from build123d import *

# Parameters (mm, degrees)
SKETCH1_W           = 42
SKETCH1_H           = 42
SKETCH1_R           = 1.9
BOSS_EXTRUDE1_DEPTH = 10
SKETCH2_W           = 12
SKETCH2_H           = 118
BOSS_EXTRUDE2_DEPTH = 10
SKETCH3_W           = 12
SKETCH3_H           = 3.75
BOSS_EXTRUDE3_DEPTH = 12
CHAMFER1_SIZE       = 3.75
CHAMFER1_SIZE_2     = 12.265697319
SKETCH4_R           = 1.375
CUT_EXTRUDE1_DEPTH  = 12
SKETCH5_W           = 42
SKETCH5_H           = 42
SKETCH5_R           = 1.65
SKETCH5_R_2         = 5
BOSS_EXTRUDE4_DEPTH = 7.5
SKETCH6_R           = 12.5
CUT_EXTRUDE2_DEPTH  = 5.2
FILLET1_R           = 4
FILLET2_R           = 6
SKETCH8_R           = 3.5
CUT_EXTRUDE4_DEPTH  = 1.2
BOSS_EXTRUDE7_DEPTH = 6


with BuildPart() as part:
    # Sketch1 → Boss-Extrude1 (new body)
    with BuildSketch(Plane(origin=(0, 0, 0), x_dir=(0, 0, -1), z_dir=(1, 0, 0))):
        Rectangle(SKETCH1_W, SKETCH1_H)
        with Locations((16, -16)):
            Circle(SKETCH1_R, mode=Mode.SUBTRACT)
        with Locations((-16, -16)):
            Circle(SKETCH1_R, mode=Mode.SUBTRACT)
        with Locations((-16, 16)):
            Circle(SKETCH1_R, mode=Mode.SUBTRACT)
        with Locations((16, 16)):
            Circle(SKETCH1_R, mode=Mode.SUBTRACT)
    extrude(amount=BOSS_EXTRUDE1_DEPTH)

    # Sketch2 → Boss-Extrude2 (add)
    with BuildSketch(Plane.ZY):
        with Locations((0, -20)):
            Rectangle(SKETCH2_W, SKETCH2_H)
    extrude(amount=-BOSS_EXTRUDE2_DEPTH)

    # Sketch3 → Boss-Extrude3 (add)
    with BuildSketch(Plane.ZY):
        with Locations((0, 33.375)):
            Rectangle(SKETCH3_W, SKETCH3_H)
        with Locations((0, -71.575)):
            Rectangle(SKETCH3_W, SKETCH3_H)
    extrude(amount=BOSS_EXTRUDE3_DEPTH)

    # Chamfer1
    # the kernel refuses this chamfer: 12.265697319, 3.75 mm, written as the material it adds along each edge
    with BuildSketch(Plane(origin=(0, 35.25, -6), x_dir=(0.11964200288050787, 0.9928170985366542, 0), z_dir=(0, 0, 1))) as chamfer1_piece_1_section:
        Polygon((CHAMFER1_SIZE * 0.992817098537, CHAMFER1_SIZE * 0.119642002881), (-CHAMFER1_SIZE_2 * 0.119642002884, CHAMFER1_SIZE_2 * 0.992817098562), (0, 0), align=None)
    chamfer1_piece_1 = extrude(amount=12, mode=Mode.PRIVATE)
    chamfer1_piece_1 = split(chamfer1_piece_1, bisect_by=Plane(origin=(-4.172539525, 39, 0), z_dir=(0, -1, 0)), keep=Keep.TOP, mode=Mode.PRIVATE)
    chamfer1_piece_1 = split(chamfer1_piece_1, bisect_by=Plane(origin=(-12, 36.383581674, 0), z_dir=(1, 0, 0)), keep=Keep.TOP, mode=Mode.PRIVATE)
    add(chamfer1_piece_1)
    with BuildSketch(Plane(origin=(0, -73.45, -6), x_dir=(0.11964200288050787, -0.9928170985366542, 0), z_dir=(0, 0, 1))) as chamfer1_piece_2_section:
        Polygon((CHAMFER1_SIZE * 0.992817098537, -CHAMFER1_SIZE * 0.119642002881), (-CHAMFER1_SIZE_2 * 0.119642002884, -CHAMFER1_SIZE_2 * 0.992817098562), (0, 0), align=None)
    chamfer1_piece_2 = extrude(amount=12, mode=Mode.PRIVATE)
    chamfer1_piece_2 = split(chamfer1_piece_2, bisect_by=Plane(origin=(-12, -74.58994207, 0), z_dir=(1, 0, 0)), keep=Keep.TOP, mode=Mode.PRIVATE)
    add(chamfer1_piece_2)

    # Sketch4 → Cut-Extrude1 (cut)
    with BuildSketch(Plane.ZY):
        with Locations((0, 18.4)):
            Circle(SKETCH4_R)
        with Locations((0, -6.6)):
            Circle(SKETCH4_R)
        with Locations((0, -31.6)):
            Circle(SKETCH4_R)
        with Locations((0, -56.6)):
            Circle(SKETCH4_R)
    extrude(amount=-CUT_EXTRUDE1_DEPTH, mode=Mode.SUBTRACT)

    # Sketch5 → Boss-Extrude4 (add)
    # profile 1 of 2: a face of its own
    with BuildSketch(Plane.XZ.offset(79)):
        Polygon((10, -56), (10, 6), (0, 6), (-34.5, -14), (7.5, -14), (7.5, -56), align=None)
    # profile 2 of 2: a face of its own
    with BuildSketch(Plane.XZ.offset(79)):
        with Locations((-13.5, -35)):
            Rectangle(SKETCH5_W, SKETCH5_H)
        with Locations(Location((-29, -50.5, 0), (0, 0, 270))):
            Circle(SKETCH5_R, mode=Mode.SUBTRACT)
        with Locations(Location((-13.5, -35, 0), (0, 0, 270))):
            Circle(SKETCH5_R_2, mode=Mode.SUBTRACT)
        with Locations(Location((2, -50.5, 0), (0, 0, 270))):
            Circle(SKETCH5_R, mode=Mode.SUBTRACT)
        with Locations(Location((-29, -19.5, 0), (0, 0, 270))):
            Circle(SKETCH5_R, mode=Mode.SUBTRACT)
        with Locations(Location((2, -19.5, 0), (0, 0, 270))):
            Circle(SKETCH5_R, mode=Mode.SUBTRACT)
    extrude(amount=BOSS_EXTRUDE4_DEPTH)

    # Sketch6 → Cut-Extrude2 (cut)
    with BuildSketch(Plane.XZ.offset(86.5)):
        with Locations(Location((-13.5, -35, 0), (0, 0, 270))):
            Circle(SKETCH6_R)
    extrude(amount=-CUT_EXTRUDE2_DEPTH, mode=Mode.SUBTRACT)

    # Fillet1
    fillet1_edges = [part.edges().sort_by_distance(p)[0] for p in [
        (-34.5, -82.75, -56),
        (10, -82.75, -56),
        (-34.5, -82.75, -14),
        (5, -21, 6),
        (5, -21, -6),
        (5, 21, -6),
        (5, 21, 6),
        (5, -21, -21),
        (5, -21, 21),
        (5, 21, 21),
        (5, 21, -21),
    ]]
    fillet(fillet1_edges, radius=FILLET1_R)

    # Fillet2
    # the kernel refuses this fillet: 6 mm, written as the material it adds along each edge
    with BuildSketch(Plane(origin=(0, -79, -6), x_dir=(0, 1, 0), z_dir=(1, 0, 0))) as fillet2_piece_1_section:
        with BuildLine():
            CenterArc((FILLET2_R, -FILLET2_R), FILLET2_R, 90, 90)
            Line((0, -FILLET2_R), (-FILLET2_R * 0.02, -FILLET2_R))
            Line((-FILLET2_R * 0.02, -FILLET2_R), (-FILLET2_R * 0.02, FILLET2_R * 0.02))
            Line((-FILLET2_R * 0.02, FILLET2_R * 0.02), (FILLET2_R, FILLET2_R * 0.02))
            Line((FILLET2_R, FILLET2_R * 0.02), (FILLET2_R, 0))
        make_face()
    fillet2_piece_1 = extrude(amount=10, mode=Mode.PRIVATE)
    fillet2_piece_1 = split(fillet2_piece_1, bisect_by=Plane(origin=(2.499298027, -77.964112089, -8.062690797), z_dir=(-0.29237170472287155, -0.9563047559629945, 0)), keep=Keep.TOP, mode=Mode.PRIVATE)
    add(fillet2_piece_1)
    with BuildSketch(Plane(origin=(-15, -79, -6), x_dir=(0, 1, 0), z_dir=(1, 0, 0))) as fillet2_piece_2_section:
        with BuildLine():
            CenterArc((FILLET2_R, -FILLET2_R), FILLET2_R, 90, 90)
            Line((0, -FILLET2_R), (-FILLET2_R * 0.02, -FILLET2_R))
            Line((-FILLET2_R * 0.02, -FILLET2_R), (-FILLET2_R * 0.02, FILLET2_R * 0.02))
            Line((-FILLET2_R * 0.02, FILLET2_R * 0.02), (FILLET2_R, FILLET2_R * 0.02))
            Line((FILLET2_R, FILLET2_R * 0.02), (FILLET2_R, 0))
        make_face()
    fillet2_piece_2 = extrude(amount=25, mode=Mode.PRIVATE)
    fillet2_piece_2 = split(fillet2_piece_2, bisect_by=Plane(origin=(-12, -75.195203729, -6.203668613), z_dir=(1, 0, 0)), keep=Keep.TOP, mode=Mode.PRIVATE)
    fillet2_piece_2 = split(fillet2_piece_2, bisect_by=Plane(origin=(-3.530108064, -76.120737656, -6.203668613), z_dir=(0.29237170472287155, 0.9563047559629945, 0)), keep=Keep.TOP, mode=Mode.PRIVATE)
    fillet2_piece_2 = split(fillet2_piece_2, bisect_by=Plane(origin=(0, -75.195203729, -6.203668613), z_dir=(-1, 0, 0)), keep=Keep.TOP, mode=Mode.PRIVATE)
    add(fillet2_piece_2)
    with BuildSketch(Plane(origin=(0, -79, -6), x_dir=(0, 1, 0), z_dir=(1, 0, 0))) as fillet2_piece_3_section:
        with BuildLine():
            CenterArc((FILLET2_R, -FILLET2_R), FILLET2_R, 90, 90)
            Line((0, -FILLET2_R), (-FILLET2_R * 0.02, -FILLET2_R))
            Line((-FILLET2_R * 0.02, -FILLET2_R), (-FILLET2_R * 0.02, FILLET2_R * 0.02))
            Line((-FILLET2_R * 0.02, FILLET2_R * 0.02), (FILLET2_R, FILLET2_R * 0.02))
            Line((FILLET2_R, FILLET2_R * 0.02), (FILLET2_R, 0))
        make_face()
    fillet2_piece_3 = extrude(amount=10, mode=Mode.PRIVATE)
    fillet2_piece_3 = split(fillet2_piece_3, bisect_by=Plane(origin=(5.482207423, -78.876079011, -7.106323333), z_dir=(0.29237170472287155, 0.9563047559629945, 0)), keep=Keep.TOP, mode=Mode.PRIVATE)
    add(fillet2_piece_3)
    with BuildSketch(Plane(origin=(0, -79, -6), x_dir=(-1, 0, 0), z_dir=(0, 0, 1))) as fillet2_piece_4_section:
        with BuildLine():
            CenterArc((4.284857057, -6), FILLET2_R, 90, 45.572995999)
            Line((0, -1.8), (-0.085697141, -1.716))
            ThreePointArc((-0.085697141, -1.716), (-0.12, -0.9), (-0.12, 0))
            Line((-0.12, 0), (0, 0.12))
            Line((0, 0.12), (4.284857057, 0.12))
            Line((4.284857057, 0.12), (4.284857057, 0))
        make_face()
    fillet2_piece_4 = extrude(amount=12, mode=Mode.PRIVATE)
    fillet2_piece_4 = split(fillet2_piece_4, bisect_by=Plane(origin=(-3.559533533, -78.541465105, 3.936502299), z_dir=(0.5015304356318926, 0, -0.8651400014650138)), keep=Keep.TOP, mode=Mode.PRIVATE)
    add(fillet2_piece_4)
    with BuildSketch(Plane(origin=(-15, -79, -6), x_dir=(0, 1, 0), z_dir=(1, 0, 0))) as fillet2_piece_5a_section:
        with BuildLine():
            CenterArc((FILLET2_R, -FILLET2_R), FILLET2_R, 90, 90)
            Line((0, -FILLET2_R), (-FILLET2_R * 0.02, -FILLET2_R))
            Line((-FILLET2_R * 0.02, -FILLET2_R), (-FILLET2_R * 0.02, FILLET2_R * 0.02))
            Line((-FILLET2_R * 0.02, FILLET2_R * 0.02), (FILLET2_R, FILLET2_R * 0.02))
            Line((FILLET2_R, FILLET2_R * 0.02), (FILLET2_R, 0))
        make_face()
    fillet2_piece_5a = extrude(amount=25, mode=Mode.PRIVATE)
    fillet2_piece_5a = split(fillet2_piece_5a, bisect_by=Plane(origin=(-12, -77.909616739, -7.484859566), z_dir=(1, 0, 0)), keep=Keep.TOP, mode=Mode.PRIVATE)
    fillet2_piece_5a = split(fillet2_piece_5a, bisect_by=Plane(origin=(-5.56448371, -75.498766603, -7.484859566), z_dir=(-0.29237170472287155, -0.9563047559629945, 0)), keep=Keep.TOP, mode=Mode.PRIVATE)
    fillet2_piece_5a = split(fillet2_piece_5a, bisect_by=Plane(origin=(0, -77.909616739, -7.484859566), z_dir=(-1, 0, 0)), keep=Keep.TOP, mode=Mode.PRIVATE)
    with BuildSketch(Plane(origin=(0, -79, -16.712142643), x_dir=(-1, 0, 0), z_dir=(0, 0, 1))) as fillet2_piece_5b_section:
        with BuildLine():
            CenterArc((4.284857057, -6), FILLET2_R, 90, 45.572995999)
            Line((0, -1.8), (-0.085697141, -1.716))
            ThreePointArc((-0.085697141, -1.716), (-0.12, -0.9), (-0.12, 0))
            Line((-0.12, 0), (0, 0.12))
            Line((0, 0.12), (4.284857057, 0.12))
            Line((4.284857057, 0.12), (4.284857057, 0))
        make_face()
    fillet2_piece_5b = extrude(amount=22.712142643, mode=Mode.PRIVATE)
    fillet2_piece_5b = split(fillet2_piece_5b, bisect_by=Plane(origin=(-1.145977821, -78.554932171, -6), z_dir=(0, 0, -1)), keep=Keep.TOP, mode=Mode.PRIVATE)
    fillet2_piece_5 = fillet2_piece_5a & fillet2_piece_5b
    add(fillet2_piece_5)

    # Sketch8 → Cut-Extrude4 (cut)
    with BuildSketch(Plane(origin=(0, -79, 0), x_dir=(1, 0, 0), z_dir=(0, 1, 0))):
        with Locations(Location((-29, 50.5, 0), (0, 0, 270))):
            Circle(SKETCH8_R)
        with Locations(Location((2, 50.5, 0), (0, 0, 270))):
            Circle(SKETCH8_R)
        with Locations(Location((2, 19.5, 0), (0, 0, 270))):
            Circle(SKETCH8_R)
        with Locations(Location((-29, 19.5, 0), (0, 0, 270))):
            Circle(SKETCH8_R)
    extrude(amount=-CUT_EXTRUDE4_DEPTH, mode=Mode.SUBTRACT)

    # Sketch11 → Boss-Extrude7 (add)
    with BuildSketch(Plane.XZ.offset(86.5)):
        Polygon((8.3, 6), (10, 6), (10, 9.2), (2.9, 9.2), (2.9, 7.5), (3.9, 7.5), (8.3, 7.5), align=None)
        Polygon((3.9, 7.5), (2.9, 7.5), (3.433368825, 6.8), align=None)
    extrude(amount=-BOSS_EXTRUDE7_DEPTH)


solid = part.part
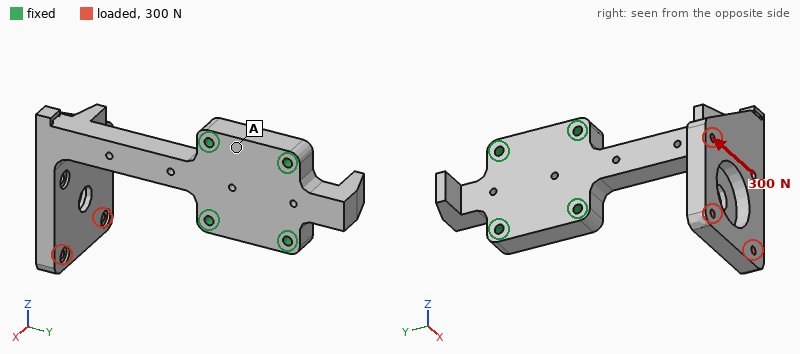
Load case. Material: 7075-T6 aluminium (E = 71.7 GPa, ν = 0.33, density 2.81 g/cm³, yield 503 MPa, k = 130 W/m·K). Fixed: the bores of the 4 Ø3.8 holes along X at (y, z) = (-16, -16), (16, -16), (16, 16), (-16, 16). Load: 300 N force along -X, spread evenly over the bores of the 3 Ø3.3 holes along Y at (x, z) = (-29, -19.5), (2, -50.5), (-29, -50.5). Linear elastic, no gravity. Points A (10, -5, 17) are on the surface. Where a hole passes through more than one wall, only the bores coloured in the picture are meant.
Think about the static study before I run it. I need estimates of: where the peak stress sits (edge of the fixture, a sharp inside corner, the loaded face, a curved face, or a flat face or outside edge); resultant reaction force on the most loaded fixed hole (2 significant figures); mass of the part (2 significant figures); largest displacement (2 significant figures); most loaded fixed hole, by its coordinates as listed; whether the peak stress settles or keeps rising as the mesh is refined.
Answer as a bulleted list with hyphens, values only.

- a sharp inside corner
- 820 N
- 120 g
- 1.4 mm
- (-16, -16)
- keeps rising
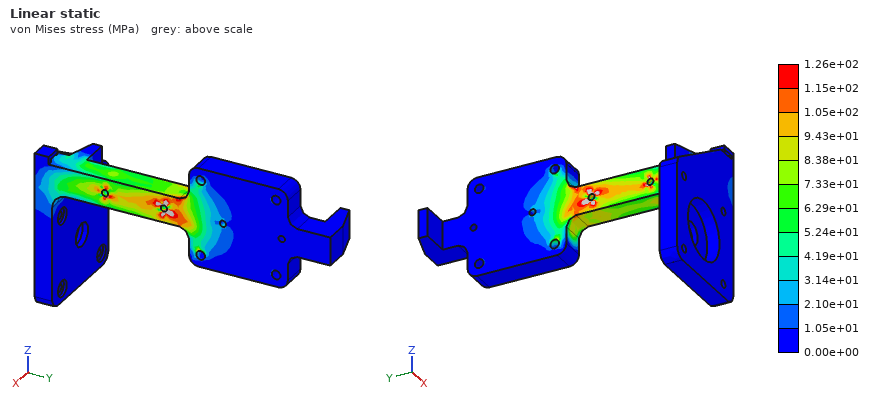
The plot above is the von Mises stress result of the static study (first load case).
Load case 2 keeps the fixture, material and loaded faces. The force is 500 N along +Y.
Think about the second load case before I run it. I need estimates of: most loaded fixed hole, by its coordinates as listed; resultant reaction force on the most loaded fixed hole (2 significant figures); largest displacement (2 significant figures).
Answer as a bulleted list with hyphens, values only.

- (-16, -16)
- 710 N
- 1.6 mm
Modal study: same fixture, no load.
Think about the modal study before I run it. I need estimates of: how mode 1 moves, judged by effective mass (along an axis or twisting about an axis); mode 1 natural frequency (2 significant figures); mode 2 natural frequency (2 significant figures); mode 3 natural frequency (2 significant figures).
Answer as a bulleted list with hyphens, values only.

- along X
- 440 Hz
- 570 Hz
- 1200 Hz
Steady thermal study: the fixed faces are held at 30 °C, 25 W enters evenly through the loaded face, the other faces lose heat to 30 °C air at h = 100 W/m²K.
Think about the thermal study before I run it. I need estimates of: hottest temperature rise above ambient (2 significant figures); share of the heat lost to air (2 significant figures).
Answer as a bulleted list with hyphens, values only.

- 39 K
- 87 %
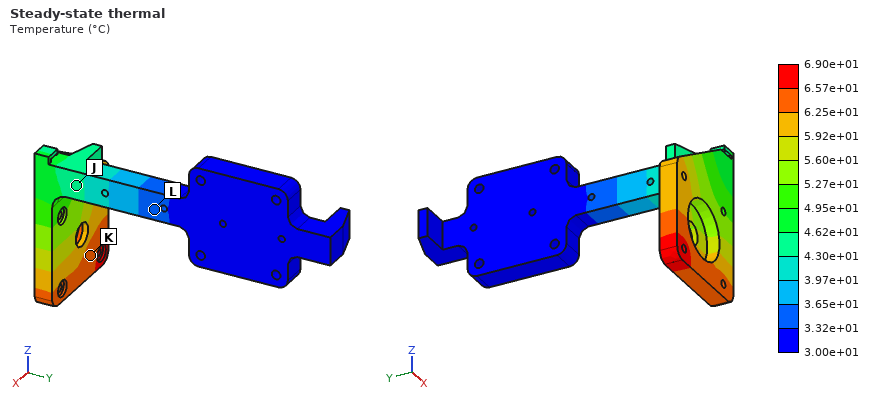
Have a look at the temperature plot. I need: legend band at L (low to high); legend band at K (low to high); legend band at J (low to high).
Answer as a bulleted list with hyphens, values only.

- 3.32e+01 to 3.65e+01 °C
- 6.25e+01 to 6.57e+01 °C
- 4.30e+01 to 4.62e+01 °C
